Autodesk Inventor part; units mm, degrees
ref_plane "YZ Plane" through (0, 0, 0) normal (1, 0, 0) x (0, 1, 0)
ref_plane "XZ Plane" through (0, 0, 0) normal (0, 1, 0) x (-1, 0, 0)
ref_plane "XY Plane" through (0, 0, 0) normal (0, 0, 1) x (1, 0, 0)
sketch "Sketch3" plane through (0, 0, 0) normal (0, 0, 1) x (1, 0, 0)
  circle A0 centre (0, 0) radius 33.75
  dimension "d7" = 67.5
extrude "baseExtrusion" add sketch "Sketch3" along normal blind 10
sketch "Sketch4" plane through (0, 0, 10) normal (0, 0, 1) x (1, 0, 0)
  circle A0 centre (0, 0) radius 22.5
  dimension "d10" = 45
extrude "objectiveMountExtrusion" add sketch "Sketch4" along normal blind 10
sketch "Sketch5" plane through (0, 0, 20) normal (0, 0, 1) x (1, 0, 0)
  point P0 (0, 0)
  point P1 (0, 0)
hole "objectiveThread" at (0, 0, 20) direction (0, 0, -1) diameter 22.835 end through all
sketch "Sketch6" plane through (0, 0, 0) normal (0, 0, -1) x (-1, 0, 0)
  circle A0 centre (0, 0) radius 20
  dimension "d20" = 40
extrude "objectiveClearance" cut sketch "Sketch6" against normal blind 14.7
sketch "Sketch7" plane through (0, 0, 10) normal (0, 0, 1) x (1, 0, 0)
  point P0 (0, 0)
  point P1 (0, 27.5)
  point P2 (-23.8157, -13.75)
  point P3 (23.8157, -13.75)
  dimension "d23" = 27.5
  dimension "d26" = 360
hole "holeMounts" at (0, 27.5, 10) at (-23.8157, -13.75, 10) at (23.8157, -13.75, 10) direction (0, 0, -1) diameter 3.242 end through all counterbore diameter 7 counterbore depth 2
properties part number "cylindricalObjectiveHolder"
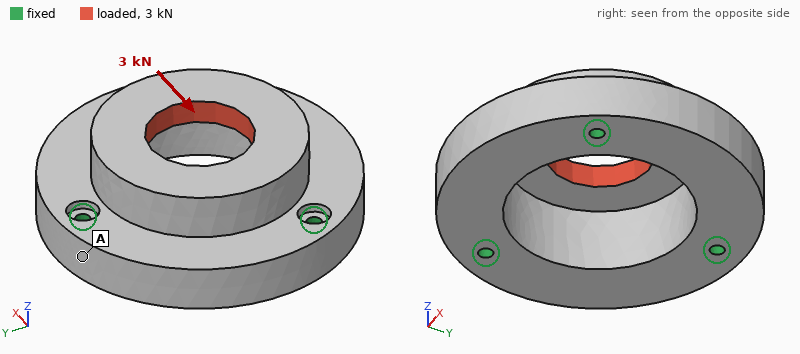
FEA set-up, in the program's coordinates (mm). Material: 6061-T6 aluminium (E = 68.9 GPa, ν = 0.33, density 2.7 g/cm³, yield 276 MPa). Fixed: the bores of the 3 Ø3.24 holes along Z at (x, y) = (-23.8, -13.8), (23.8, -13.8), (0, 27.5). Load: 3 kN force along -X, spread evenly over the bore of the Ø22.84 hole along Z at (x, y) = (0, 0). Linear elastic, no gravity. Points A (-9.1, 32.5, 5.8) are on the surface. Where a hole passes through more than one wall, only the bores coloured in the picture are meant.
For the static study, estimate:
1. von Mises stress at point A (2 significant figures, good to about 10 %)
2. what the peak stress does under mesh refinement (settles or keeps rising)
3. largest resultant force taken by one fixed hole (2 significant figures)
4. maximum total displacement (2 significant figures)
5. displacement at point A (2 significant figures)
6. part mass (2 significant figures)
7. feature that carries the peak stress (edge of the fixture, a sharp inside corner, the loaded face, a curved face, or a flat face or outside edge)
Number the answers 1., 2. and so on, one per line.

1. 4.4 MPa
2. keeps rising
3. 1.2 kN
4. 14 µm
5. 2.9 µm
6. 83 g
7. edge of the fixture
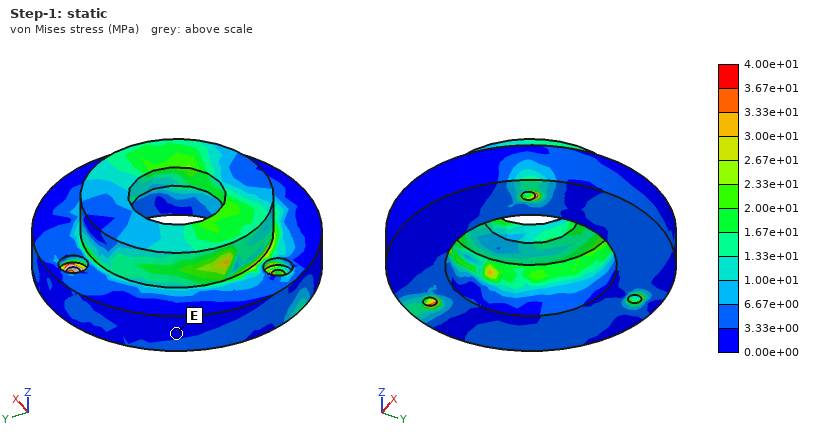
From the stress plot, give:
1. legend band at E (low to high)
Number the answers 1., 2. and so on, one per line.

1. 0.00e+00 to 3.33e+00 MPa
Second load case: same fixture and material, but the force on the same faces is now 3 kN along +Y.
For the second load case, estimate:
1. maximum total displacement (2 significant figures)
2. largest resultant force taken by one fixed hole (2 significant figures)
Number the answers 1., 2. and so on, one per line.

1. 16 µm
2. 1.2 kN
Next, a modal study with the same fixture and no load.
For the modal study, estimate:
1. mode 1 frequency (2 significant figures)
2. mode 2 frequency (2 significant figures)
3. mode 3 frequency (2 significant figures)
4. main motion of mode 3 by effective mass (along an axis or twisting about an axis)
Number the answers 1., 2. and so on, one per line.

1. 11 kHz
2. 11 kHz
3. 13 kHz
4. along Z
